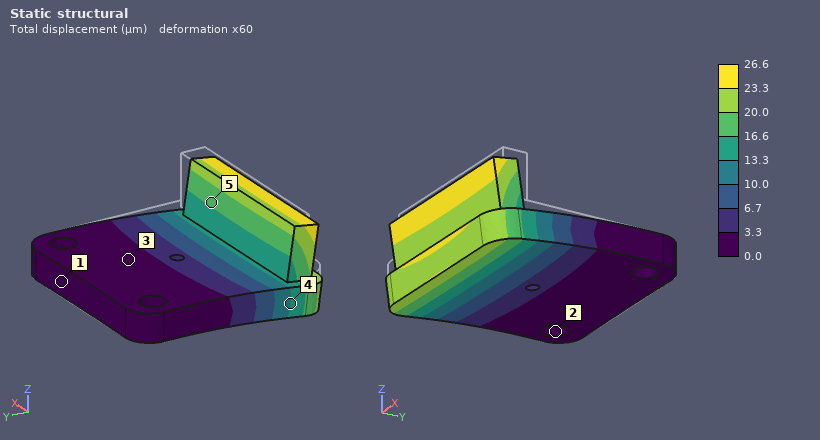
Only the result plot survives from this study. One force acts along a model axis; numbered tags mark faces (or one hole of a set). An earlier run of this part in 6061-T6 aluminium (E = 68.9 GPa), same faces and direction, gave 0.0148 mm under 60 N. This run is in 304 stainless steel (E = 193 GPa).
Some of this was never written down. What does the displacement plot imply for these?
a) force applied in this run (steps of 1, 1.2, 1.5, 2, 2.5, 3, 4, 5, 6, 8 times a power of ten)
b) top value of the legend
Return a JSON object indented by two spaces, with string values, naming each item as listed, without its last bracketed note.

{
  "force applied in this run": "300 N",
  "top value of the legend": "26.6 µm"
}
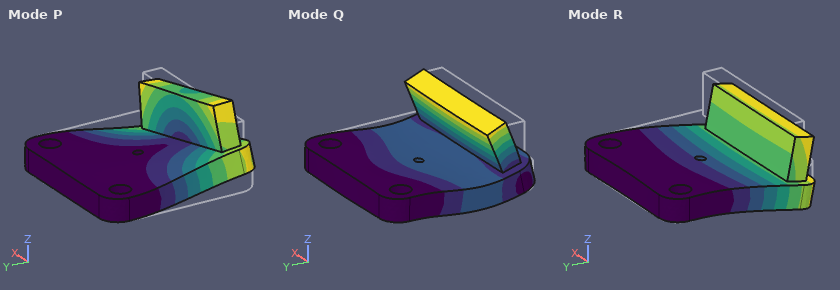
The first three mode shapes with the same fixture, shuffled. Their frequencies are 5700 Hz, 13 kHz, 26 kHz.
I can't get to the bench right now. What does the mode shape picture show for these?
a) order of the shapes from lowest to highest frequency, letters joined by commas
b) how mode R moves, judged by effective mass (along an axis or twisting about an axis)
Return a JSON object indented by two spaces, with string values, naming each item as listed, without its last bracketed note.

{
  "order of the shapes from lowest to highest frequency, letters joined by commas": "R, P, Q",
  "how mode R moves, judged by effective mass": "along Z"
}
